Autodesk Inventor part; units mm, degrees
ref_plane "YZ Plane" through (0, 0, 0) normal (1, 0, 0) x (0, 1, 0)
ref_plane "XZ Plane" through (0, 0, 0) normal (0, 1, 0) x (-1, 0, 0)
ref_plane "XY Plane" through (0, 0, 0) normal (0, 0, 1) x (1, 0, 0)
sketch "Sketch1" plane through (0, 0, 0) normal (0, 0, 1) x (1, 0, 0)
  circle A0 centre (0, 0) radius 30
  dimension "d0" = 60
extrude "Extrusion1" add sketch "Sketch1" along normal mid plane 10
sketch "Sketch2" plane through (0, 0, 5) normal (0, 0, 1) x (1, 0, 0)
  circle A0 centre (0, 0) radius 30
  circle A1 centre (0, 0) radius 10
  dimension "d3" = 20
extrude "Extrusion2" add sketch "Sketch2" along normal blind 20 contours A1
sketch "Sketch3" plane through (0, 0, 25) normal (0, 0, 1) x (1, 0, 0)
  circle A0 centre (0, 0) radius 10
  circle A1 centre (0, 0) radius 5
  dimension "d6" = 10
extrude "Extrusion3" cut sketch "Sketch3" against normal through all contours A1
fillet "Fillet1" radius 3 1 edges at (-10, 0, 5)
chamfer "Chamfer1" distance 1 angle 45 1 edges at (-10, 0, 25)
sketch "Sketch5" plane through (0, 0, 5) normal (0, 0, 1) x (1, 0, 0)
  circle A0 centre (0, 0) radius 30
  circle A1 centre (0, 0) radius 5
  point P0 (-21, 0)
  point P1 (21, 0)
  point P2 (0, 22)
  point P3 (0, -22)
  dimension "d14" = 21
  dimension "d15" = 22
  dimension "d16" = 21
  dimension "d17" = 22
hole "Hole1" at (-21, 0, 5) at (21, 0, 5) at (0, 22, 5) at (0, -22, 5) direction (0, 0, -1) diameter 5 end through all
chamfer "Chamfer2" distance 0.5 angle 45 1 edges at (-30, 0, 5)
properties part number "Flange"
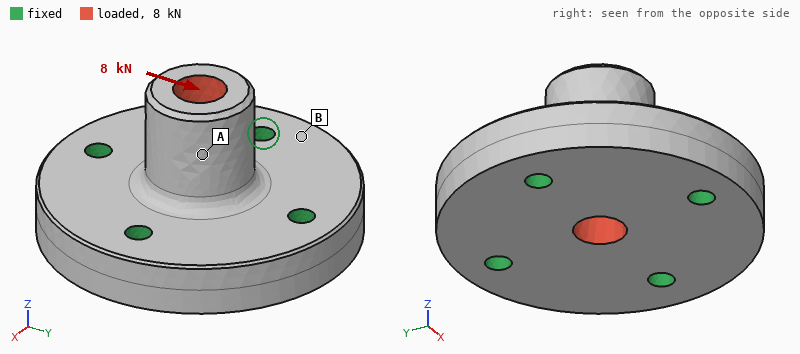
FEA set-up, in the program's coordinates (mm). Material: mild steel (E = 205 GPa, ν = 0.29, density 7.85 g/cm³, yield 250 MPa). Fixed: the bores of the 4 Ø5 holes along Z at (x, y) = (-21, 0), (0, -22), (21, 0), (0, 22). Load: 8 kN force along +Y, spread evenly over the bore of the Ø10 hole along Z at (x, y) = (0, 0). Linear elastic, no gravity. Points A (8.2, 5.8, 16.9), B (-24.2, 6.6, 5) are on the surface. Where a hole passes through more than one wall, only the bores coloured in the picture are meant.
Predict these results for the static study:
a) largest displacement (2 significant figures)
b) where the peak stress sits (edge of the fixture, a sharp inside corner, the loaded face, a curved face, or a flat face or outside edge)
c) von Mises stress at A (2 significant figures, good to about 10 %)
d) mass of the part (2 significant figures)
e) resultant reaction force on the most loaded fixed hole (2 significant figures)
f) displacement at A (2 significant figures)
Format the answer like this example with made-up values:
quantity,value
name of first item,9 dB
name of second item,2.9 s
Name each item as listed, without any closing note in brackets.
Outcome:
quantity,value
largest displacement,14 µm
where the peak stress sits,a curved face
von Mises stress at A,20 MPa
mass of the part,250 g
resultant reaction force on the most loaded fixed hole,3.2 kN
displacement at A,9.4 µm
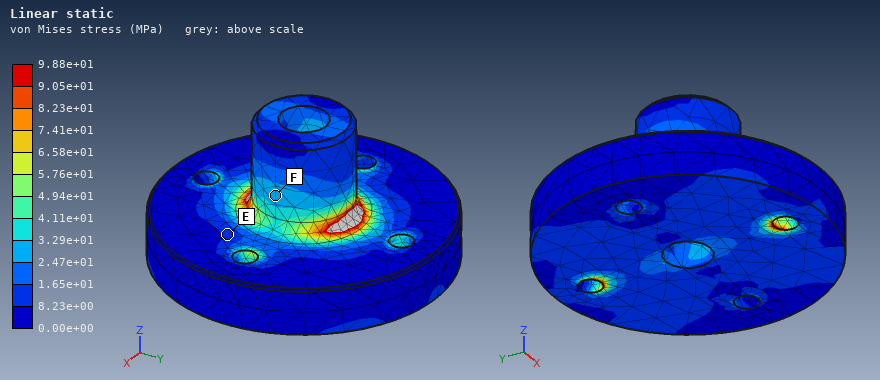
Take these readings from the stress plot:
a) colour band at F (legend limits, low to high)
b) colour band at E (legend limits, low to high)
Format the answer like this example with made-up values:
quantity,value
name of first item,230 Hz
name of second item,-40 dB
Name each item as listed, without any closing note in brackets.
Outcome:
quantity,value
colour band at F,2.47e+01 to 3.29e+01 MPa
colour band at E,8.23e+00 to 1.65e+01 MPa
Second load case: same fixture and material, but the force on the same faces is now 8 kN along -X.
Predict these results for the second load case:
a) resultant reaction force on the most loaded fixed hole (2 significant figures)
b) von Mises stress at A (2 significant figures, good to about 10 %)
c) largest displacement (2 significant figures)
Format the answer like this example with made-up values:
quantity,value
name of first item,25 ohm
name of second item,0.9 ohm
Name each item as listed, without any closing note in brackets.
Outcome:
quantity,value
resultant reaction force on the most loaded fixed hole,3.4 kN
von Mises stress at A,17 MPa
largest displacement,14 µm
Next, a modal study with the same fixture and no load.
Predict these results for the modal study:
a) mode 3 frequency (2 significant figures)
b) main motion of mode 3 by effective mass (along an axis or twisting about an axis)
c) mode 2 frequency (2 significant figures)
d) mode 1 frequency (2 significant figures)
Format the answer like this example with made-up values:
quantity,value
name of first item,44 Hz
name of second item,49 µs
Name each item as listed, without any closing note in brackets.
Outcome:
quantity,value
mode 3 frequency,25 kHz
main motion of mode 3 by effective mass,along Z
mode 2 frequency,19 kHz
mode 1 frequency,18 kHz
